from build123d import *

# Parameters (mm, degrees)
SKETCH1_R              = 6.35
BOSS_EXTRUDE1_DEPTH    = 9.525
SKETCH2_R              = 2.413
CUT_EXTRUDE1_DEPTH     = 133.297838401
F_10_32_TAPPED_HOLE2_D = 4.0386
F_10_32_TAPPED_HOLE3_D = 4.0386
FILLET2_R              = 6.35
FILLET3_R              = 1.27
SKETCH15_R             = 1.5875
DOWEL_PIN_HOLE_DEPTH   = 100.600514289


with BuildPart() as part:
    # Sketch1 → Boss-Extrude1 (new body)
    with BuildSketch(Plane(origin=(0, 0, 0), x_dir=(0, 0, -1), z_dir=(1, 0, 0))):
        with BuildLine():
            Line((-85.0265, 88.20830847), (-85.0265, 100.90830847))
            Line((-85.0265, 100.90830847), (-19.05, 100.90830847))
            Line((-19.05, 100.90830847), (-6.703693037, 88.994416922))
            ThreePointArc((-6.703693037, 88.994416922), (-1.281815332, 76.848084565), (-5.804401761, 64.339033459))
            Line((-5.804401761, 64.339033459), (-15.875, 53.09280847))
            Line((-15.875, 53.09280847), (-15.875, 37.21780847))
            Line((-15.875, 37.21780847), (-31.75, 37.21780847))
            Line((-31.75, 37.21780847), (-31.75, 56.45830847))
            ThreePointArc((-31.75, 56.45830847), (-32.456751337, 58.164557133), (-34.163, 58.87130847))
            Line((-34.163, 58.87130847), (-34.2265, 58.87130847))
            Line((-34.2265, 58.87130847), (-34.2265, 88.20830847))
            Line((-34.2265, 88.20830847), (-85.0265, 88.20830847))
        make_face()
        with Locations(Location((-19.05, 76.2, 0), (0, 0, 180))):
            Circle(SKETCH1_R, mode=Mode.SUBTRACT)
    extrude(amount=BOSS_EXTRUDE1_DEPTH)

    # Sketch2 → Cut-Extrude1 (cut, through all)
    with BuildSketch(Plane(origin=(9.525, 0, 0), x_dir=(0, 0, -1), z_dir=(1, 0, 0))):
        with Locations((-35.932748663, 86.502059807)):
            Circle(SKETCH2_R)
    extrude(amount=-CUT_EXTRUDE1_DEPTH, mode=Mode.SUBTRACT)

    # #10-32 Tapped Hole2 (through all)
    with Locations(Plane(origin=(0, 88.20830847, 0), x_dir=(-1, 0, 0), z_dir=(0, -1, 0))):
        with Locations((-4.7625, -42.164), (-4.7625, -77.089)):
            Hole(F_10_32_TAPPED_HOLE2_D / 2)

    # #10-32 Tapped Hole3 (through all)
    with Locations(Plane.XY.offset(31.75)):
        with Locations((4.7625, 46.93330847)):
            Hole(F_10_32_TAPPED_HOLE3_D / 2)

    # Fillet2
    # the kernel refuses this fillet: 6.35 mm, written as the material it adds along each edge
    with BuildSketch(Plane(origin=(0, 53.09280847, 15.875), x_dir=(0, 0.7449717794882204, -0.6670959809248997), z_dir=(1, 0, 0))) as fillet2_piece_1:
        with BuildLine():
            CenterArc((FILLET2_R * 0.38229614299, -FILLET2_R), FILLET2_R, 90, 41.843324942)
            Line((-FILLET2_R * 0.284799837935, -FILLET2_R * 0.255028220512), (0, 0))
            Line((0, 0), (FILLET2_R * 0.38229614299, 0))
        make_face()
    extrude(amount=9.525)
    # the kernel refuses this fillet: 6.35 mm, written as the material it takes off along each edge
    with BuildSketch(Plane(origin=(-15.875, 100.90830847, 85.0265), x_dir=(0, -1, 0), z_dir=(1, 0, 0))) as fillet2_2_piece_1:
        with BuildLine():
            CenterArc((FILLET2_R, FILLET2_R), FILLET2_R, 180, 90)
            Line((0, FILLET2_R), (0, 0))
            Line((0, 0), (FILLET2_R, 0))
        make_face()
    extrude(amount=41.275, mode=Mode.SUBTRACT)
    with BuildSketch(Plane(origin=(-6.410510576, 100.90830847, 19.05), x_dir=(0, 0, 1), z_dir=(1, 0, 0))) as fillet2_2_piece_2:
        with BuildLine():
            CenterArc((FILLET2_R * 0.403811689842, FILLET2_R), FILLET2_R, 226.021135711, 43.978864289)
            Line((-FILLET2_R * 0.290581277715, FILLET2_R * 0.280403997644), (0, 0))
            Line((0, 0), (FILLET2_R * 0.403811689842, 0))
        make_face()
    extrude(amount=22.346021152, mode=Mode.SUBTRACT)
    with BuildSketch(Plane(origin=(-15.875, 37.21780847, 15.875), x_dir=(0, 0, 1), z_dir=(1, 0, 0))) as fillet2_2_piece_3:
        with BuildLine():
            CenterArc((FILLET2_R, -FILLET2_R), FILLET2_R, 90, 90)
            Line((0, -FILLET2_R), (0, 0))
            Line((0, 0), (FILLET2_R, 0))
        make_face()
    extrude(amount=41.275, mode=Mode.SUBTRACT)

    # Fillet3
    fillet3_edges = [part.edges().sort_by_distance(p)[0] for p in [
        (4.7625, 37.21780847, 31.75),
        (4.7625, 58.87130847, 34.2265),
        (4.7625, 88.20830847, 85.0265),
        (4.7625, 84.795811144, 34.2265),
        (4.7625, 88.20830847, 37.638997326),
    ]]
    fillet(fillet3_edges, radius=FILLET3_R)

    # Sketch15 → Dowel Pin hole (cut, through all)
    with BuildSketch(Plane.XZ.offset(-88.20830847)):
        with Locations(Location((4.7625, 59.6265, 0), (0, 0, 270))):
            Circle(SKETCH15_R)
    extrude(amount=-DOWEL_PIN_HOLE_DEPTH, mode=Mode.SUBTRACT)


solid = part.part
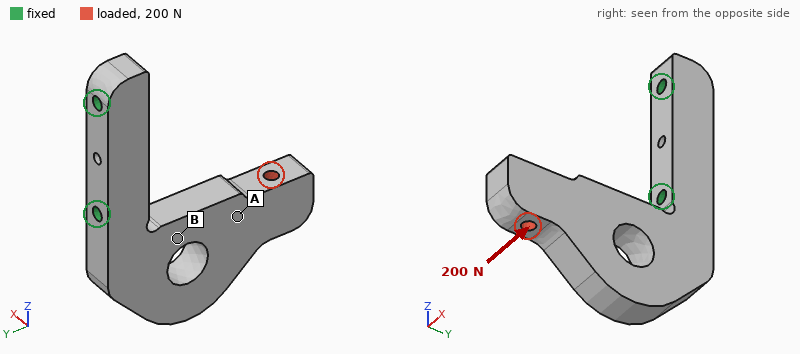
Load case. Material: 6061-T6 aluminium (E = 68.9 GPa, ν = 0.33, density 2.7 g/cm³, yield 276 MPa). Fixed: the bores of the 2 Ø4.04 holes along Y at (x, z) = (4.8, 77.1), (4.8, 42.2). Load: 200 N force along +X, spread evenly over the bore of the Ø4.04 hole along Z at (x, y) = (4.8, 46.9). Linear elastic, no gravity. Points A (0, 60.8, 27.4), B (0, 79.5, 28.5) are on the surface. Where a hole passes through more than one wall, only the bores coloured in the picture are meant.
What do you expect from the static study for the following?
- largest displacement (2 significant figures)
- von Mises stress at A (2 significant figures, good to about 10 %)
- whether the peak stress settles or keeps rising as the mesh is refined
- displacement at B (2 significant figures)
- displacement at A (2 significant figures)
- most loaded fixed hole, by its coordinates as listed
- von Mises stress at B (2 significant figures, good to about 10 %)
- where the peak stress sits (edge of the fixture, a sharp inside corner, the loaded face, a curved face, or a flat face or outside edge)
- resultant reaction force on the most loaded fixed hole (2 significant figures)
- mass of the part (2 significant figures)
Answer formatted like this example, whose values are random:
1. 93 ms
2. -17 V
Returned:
1. 0.23 mm
2. 9.6 MPa
3. keeps rising
4. 0.047 mm
5. 0.12 mm
6. (4.8, 42.2)
7. 29 MPa
8. edge of the fixture
9. 220 N
10. 50 g
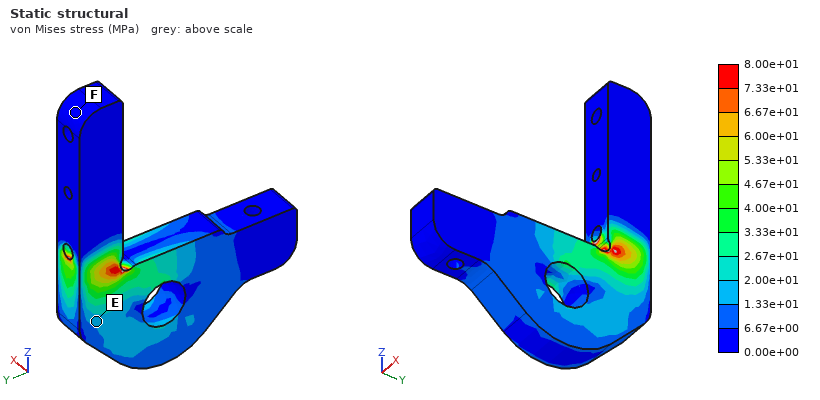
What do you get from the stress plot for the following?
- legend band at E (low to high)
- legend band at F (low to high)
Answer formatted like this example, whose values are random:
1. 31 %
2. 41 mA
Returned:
1. 1.33e+01 to 2.00e+01 MPa
2. 0.00e+00 to 6.67e+00 MPa
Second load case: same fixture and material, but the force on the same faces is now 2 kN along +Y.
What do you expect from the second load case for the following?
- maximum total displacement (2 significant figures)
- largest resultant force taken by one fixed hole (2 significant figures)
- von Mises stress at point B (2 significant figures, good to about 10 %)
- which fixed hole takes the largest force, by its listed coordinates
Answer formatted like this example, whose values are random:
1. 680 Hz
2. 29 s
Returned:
1. 0.19 mm
2. 2.1 kN
3. 16 MPa
4. (4.8, 42.2)
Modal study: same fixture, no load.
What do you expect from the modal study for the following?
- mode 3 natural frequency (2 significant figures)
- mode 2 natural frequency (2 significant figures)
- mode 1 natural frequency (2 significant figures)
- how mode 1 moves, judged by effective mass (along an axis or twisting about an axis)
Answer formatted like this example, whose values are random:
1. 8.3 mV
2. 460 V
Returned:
1. 3700 Hz
2. 2100 Hz
3. 1500 Hz
4. along X
